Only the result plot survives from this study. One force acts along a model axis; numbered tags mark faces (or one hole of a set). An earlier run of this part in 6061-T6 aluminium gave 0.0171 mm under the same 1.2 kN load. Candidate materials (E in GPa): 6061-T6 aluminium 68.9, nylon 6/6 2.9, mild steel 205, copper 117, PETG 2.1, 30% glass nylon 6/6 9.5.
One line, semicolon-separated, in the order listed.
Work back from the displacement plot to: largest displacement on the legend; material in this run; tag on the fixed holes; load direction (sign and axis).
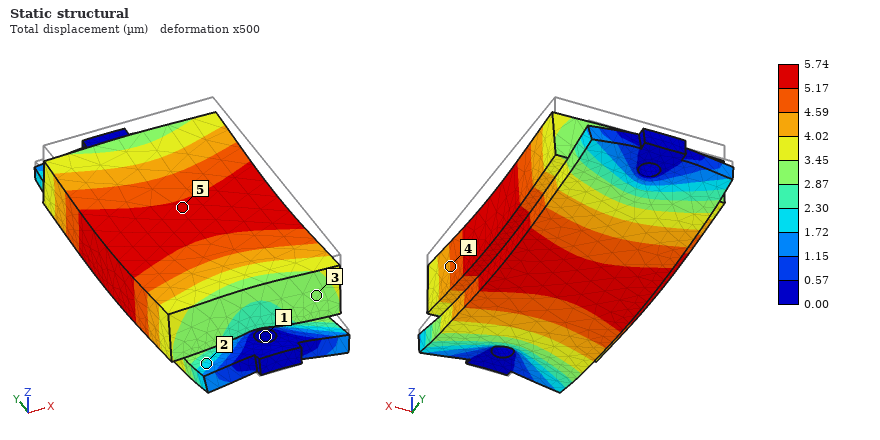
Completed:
5.74 µm; mild steel; 1; -Z
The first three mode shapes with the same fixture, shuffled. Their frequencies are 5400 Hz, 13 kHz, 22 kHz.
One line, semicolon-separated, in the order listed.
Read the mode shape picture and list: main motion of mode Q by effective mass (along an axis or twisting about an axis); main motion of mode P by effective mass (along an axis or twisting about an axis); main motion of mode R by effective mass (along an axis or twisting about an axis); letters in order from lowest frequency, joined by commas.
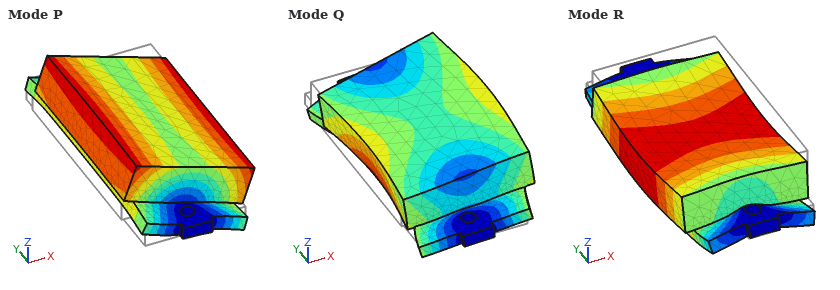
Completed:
along X; along X; along Z; P, R, Q
